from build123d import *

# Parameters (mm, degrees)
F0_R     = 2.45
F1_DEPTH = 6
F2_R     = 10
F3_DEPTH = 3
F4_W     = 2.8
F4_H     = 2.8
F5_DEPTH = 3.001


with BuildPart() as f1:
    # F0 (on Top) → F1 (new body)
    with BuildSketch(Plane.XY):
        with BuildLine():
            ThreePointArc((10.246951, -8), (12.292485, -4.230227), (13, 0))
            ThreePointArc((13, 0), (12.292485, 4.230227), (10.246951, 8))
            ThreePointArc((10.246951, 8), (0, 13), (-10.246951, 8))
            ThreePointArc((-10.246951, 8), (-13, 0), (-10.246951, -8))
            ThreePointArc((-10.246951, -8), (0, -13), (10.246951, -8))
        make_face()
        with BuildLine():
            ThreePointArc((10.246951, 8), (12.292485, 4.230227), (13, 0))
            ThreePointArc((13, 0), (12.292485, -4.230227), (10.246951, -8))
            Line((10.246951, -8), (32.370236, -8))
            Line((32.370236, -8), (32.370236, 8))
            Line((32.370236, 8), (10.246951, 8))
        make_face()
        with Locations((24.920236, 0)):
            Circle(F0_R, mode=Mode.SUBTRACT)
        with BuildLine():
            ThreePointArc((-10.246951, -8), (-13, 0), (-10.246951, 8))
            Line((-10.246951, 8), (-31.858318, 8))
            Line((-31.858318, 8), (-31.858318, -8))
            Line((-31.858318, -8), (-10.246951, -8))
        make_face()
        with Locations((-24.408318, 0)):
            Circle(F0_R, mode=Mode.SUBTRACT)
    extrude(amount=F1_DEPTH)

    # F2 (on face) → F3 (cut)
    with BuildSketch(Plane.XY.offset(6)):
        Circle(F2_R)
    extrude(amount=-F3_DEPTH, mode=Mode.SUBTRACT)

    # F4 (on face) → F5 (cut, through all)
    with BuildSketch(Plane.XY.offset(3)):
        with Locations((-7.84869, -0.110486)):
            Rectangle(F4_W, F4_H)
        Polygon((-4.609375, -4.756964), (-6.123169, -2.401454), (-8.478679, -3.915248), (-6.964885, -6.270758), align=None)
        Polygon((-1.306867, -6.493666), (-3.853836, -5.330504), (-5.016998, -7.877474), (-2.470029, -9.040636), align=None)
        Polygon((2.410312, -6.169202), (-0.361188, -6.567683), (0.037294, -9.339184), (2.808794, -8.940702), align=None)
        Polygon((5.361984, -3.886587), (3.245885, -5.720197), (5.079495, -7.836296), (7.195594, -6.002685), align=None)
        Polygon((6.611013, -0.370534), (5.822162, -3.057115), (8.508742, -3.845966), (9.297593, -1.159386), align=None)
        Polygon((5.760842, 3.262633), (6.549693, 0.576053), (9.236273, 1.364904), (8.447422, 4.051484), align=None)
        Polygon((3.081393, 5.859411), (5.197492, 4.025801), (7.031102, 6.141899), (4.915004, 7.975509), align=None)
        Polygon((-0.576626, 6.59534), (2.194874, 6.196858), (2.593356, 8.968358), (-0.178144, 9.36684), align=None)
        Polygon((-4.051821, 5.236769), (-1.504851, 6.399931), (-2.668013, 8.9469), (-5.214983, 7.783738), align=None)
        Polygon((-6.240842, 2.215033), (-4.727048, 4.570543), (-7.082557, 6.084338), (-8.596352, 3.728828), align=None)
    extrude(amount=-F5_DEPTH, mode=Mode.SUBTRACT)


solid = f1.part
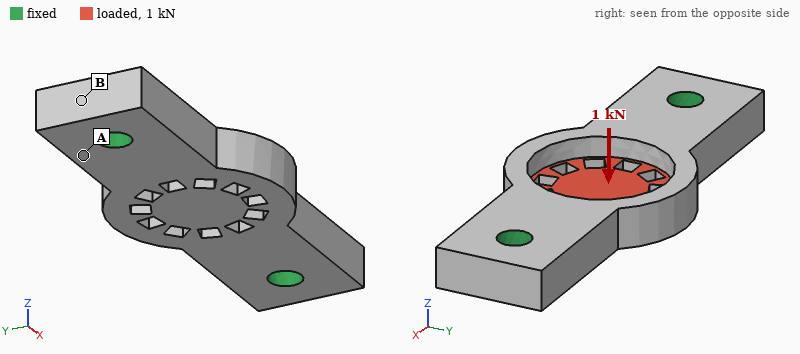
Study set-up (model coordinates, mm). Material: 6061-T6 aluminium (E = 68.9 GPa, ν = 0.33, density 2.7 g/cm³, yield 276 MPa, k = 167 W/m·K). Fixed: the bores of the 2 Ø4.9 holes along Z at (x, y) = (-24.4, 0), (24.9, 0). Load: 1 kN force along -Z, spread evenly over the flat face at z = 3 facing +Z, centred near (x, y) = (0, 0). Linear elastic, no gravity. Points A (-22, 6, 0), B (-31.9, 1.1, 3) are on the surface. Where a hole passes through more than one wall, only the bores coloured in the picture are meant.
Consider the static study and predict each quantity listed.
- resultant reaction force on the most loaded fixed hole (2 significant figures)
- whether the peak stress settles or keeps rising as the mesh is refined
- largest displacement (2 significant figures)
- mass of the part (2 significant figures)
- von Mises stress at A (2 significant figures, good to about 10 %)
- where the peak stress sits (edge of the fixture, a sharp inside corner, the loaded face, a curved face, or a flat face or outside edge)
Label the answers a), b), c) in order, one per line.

a) 610 N
b) keeps rising
c) 45 µm
d) 15 g
e) 32 MPa
f) edge of the fixture
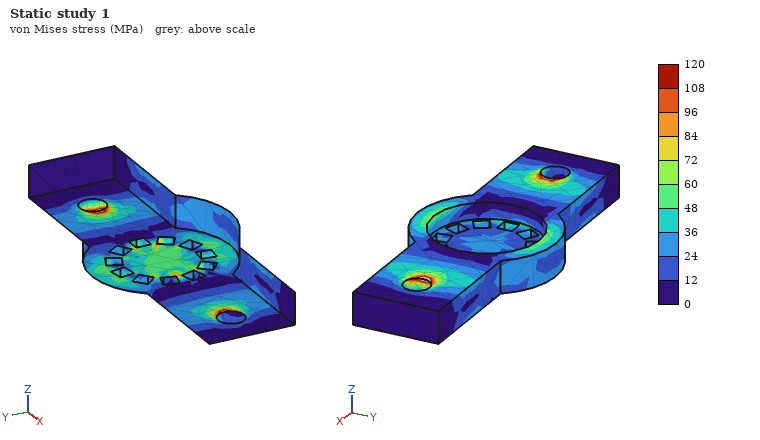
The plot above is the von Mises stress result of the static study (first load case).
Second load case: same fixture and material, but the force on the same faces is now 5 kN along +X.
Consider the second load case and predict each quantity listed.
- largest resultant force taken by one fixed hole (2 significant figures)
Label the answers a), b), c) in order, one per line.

a) 2.5 kN
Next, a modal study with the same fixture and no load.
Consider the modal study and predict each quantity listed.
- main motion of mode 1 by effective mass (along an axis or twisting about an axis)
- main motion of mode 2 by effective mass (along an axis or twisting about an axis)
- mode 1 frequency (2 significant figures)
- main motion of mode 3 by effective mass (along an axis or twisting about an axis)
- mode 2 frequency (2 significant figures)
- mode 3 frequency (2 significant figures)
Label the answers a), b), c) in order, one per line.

a) along Z
b) twisting about X
c) 11 kHz
d) along Y
e) 14 kHz
f) 21 kHz
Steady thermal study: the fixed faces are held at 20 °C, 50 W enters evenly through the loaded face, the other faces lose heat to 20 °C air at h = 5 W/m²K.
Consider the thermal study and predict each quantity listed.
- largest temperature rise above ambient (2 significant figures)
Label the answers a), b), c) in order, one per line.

a) 49 K
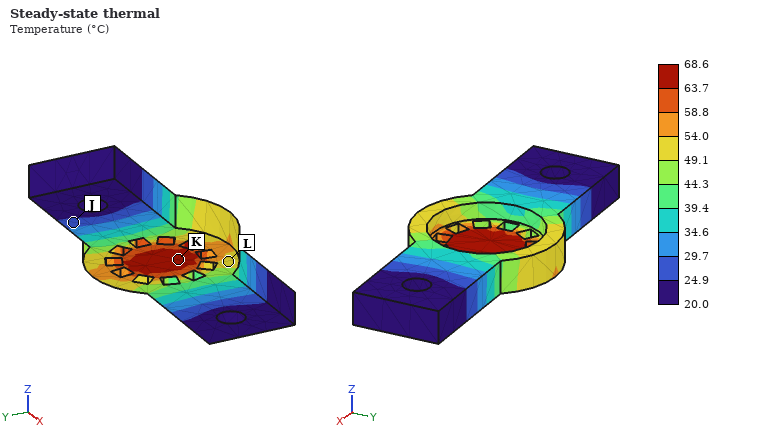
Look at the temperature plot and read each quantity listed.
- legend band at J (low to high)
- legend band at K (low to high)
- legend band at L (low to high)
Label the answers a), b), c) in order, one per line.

a) 24.9 to 29.7 °C
b) 63.7 to 68.6 °C
c) 49.1 to 54.0 °C
